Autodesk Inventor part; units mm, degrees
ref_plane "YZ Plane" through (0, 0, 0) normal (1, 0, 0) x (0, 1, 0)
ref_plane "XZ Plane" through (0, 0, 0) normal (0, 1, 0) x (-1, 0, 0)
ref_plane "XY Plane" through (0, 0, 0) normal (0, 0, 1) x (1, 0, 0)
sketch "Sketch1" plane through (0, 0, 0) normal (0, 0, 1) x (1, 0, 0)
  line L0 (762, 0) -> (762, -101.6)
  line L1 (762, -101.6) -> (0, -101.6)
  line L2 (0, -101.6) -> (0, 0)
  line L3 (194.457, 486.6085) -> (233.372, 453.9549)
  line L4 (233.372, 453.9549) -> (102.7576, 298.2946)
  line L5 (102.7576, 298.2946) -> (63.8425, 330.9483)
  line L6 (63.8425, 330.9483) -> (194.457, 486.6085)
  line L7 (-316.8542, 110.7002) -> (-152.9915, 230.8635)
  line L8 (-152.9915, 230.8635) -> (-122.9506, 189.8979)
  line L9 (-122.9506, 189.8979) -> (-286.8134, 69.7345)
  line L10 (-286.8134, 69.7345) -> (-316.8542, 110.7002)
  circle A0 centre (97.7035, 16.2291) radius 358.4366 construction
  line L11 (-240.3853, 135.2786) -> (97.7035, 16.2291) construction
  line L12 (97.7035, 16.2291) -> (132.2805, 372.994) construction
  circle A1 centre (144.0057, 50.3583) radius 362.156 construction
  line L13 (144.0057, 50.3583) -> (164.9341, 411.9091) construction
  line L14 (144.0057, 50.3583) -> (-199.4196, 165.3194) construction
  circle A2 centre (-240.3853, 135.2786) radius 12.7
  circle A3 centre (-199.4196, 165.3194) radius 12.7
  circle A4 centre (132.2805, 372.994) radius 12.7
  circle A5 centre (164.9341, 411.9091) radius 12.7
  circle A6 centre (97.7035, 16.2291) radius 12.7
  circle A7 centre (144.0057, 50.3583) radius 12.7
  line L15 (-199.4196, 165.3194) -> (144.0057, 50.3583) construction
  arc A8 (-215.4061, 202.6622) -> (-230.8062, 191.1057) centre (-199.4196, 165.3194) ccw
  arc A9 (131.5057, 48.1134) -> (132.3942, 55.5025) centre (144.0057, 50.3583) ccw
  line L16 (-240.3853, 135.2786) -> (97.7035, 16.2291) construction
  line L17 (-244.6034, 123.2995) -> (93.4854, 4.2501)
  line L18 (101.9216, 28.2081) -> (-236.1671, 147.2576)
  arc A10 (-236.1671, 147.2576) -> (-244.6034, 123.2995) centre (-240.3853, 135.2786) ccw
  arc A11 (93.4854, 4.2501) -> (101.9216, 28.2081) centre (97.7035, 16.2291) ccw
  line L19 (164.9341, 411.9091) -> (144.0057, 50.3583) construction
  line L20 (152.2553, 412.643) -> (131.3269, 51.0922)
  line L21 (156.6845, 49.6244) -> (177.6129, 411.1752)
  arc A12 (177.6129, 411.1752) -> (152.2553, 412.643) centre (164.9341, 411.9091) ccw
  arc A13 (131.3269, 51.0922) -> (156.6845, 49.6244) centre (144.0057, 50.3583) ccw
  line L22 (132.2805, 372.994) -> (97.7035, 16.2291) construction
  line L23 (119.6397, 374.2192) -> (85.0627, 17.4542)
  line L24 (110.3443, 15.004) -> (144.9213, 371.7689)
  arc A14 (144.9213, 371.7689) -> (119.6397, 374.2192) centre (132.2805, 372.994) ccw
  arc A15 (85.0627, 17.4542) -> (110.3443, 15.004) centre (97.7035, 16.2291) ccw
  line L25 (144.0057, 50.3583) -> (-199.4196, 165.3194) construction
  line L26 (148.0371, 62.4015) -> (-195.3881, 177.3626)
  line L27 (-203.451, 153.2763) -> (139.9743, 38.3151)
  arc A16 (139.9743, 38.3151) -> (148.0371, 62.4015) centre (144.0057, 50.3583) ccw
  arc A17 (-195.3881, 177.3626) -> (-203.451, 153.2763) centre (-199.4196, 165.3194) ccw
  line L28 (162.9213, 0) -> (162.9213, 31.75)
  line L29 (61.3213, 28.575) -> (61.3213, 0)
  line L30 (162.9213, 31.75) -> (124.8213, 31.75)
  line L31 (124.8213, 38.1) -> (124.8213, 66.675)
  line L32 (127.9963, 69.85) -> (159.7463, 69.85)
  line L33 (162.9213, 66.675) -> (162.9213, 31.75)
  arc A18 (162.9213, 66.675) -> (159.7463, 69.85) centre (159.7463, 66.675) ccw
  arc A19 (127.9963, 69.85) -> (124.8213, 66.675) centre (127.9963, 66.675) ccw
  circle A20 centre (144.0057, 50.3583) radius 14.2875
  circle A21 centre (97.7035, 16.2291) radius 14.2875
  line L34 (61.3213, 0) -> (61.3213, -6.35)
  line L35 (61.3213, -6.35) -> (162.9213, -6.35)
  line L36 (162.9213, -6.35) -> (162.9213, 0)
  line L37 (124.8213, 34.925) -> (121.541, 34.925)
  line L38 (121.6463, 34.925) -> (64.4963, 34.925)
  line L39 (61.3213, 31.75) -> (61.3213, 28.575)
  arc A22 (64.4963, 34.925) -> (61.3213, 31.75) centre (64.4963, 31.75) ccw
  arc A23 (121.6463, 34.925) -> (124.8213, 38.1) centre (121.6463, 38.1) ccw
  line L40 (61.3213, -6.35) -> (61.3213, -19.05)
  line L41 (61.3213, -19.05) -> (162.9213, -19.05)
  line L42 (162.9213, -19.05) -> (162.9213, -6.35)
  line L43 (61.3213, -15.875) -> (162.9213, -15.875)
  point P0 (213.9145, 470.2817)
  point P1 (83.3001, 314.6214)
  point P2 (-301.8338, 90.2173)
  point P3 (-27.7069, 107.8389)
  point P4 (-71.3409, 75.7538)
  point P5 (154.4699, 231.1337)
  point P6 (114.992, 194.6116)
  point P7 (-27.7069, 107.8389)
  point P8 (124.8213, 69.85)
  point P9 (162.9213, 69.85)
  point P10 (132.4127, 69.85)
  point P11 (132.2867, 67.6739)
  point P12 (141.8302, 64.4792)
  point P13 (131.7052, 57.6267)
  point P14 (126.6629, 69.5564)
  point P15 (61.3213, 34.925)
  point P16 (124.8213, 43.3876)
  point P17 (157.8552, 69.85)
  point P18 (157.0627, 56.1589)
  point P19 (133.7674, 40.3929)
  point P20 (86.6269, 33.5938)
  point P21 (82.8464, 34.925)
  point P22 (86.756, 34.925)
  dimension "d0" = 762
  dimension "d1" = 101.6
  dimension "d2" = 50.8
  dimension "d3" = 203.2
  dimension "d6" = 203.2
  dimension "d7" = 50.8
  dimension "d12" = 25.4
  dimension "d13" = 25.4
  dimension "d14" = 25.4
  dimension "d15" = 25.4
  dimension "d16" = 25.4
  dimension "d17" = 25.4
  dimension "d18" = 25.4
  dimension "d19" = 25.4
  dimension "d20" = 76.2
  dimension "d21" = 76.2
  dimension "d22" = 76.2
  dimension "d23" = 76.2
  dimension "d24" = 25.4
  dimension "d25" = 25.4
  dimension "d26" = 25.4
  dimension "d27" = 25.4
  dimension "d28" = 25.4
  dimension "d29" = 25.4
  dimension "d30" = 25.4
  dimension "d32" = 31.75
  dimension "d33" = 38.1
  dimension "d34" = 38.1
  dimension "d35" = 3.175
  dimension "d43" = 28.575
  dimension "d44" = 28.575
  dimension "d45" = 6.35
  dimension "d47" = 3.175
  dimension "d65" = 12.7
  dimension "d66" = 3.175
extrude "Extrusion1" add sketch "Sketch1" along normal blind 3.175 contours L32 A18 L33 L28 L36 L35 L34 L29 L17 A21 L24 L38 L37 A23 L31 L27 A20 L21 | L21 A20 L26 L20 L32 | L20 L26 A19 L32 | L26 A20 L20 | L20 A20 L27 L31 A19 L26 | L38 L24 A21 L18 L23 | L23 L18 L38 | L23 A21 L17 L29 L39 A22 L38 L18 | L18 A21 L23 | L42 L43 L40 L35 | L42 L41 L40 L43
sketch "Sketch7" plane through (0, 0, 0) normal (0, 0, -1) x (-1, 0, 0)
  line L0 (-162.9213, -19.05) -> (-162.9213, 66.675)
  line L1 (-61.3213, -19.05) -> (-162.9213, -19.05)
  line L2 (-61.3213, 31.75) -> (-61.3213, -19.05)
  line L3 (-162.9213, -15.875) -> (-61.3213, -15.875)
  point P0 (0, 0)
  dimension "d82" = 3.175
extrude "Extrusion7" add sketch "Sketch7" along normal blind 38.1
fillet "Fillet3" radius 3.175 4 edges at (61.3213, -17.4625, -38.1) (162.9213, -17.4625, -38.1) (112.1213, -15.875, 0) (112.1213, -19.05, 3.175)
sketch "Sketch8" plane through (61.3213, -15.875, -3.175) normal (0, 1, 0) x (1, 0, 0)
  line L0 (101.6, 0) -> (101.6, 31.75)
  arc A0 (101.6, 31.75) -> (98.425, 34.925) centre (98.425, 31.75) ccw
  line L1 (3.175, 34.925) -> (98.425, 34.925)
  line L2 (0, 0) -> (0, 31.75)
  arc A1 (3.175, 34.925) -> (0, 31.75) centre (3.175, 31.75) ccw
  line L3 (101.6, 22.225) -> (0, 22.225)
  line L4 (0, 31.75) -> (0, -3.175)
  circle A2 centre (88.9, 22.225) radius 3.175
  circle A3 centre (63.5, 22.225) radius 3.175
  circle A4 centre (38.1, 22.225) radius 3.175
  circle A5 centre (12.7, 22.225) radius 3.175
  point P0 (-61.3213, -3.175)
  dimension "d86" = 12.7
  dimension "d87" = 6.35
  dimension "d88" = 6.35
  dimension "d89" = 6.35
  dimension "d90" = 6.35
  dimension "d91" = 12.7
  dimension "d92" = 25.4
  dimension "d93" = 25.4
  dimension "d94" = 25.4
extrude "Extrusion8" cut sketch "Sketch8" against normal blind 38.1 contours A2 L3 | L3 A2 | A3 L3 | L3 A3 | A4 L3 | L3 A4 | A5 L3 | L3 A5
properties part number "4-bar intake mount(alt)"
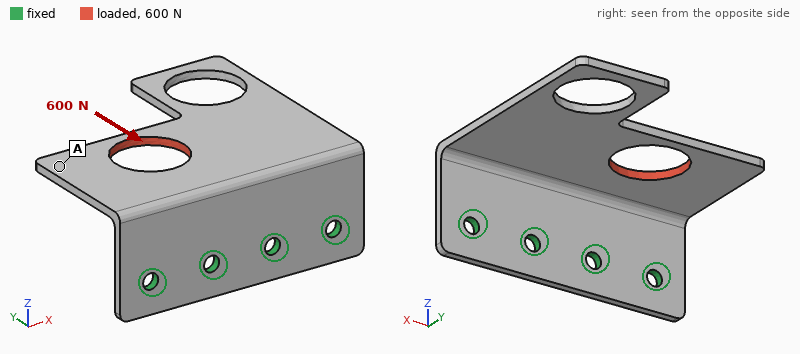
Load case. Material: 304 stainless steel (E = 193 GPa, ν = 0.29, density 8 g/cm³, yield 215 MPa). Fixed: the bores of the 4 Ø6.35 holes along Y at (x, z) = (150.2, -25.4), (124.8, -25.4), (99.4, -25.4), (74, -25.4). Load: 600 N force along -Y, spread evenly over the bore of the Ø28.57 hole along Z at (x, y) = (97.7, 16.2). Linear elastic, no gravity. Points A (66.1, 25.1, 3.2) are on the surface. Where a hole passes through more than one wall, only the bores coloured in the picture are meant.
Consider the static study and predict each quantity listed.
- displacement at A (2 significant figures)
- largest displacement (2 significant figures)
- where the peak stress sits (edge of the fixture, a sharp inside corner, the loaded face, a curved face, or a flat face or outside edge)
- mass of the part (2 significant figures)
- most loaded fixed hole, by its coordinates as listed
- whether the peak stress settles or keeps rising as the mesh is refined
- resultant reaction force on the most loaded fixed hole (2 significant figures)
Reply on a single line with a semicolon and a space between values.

0.20 mm; 0.30 mm; edge of the fixture; 240 g; (74, -25.4); keeps rising; 250 N
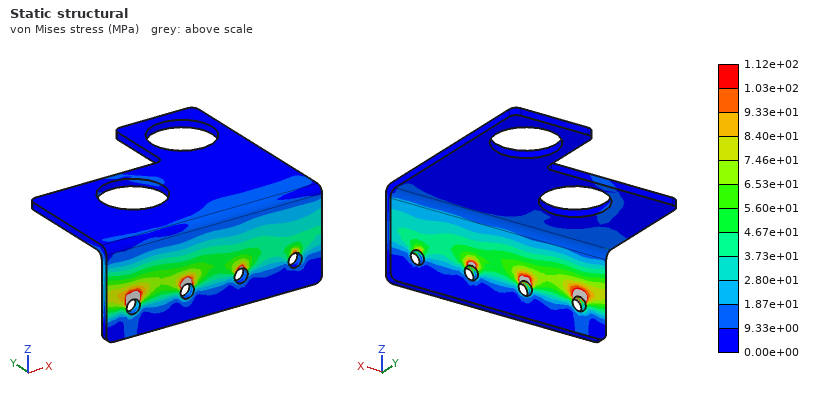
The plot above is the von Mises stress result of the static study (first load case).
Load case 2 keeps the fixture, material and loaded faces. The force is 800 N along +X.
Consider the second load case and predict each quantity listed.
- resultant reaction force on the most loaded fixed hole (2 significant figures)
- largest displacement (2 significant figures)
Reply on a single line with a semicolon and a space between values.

450 N; 0.21 mm
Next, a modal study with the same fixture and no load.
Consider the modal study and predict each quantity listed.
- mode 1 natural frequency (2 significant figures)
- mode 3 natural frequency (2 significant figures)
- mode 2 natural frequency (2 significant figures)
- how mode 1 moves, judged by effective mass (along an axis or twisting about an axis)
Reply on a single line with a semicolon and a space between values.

380 Hz; 1200 Hz; 850 Hz; along Z
